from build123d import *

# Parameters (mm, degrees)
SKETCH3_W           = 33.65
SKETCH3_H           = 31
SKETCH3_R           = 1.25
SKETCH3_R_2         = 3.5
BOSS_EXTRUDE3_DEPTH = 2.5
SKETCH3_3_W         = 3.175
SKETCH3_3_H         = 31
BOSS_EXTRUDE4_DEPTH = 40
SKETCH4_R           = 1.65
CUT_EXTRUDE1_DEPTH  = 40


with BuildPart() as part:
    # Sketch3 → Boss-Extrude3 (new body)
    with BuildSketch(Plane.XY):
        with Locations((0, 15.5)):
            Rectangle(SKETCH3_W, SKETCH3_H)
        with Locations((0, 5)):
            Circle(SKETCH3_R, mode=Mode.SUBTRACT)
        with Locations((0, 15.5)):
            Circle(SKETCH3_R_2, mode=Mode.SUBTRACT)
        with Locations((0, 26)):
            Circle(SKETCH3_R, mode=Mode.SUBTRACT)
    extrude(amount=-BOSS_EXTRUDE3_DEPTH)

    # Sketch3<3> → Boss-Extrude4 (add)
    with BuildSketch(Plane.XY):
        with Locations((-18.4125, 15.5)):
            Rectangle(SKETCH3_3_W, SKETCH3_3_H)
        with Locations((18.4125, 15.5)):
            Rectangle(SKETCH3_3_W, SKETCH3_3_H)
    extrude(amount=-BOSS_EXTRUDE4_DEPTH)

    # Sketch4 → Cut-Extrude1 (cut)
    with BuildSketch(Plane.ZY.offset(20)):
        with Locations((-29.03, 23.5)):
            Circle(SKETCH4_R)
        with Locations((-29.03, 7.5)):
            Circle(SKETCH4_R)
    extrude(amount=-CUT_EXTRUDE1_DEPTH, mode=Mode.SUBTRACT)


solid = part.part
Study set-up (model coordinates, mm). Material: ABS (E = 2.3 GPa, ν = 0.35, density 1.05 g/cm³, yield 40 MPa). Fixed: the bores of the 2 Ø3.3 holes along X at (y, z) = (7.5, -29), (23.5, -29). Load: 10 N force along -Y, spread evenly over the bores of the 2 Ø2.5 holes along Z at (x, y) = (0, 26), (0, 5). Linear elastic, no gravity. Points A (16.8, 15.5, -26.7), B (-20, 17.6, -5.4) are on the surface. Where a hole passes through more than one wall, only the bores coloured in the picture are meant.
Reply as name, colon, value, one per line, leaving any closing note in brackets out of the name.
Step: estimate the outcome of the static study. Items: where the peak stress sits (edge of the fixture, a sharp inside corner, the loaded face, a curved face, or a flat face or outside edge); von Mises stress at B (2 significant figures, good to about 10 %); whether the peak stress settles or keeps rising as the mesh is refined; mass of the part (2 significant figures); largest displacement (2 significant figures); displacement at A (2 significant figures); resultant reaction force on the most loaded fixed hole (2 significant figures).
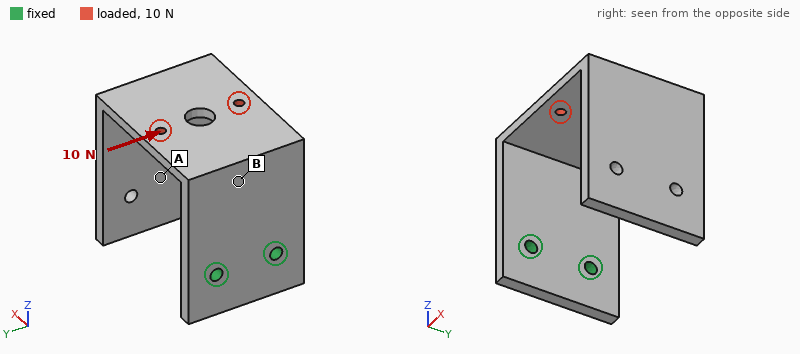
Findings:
where the peak stress sits: edge of the fixture
von Mises stress at B: 2.1 MPa
whether the peak stress settles or keeps rising as the mesh is refined: keeps rising
mass of the part: 11 g
largest displacement: 0.66 mm
displacement at A: 0.54 mm
resultant reaction force on the most loaded fixed hole: 18 N
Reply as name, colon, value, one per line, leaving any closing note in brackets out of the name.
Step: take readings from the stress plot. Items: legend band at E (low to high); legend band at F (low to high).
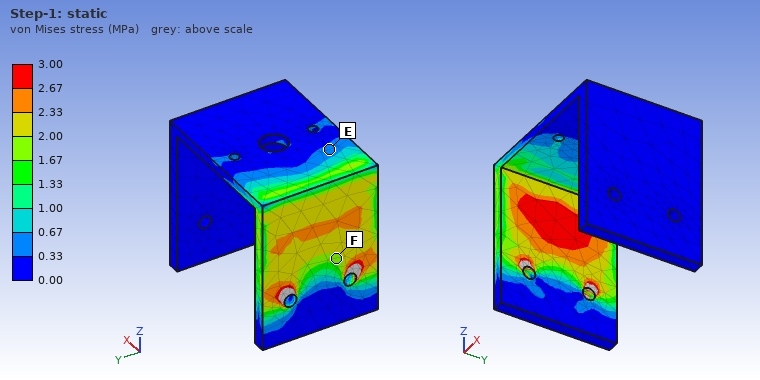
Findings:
legend band at E: 0.33 to 0.67 MPa
legend band at F: 1.67 to 2.00 MPa
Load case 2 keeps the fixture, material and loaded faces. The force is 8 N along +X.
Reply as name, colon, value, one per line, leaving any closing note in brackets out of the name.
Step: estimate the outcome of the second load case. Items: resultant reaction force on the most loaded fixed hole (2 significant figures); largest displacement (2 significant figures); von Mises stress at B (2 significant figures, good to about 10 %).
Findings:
resultant reaction force on the most loaded fixed hole: 4.0 N
largest displacement: 0.66 mm
von Mises stress at B: 0.61 MPa
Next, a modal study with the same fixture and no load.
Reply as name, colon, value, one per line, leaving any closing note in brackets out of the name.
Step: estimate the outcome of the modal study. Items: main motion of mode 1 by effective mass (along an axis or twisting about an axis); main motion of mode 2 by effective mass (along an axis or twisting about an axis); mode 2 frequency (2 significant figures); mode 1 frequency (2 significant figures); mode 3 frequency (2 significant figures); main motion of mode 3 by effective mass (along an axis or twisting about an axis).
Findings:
main motion of mode 1 by effective mass: along Z
main motion of mode 2 by effective mass: along Y
mode 2 frequency: 160 Hz
mode 1 frequency: 100 Hz
mode 3 frequency: 250 Hz
main motion of mode 3 by effective mass: along X
